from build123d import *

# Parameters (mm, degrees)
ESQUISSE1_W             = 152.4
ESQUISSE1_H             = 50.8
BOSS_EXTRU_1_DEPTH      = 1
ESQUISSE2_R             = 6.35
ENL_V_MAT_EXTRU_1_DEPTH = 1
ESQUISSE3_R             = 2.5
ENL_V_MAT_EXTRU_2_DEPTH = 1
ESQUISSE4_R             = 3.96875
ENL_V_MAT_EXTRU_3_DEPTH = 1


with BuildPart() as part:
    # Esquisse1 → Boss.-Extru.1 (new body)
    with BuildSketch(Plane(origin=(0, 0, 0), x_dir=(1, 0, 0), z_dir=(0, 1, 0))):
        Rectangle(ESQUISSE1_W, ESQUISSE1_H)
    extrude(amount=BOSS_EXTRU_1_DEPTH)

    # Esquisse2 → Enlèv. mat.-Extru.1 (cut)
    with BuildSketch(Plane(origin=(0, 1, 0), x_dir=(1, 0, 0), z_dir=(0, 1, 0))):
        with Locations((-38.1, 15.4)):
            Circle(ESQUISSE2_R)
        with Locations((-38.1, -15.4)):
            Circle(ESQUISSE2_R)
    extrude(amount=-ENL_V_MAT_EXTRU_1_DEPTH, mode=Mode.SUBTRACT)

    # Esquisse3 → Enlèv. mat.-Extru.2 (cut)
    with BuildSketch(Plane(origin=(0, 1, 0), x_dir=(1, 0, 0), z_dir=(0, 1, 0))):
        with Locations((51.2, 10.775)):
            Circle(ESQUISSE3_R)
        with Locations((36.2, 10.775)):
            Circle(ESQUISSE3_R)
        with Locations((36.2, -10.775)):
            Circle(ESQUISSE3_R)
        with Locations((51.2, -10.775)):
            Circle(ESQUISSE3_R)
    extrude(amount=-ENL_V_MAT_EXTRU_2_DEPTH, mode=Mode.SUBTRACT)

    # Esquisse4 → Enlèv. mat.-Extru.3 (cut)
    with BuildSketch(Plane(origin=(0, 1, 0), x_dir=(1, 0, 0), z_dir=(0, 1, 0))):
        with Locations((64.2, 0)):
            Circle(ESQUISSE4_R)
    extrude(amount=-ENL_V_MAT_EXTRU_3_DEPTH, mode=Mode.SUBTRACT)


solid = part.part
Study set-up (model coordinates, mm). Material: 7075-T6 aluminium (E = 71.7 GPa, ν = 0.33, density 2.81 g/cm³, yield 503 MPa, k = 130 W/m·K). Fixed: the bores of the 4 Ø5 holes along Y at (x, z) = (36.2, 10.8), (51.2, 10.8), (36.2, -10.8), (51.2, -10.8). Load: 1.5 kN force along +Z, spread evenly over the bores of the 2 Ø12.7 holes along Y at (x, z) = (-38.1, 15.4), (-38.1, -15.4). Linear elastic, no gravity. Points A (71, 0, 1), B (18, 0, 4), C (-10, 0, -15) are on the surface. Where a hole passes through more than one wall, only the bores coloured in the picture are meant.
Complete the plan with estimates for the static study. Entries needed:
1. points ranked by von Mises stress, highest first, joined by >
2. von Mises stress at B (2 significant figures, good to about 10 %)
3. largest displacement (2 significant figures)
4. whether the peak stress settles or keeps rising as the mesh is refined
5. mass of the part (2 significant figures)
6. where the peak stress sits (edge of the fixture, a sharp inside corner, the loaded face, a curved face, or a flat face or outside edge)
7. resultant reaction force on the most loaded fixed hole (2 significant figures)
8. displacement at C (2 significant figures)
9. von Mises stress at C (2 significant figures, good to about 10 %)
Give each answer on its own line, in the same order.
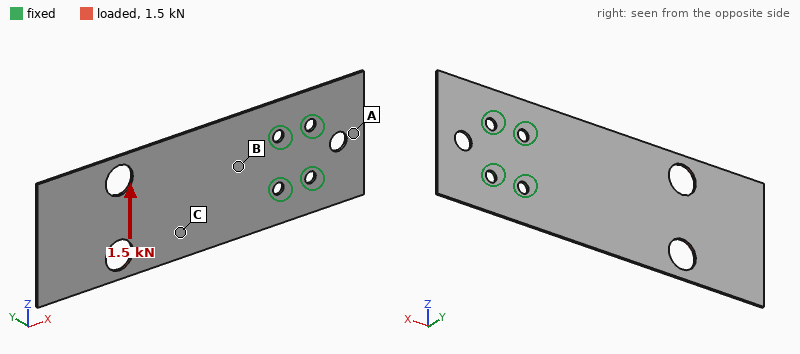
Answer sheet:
B > C > A
100 MPa
0.76 mm
keeps rising
21 g
edge of the fixture
3.0 kN
0.26 mm
77 MPa
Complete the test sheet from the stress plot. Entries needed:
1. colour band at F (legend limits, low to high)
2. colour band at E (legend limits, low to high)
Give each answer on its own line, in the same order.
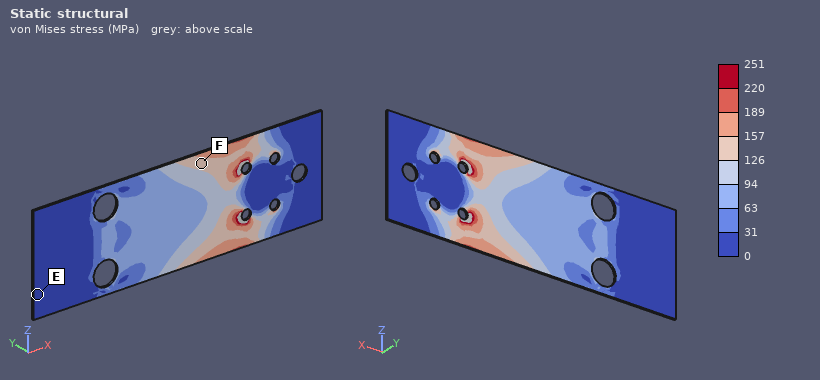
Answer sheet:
126 to 157 MPa
0 to 31 MPa
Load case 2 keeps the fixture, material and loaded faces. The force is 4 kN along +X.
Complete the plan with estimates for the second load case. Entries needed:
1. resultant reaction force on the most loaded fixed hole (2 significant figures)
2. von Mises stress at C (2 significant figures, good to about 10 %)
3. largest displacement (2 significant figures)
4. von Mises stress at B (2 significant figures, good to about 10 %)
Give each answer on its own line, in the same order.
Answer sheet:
1.6 kN
78 MPa
0.10 mm
85 MPa
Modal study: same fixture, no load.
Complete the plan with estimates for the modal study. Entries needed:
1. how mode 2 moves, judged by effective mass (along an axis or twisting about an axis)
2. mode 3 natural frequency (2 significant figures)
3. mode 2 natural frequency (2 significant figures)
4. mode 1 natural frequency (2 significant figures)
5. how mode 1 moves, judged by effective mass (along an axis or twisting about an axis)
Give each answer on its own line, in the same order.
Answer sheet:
twisting about X
400 Hz
310 Hz
69 Hz
along Y
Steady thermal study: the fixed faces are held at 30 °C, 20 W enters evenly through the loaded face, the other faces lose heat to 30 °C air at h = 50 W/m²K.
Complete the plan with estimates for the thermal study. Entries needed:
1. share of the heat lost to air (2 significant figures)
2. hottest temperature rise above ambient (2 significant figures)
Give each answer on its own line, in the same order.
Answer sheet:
86 %
67 K
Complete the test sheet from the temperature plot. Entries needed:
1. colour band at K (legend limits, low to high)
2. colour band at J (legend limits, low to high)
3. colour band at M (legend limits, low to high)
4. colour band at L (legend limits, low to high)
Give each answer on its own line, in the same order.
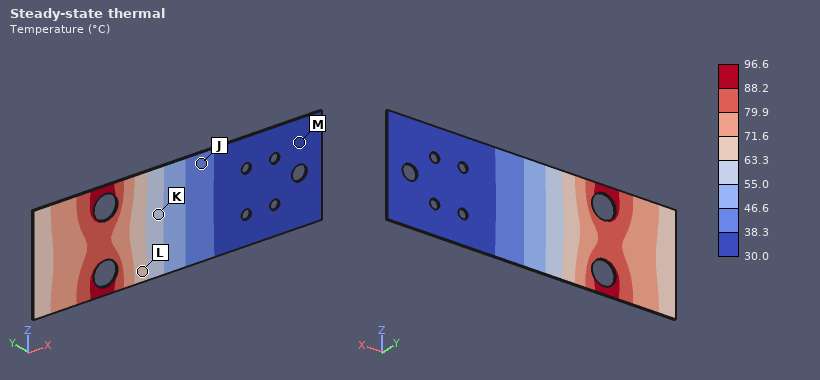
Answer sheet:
55.0 to 63.3 °C
38.3 to 46.6 °C
30.0 to 38.3 °C
63.3 to 71.6 °C
